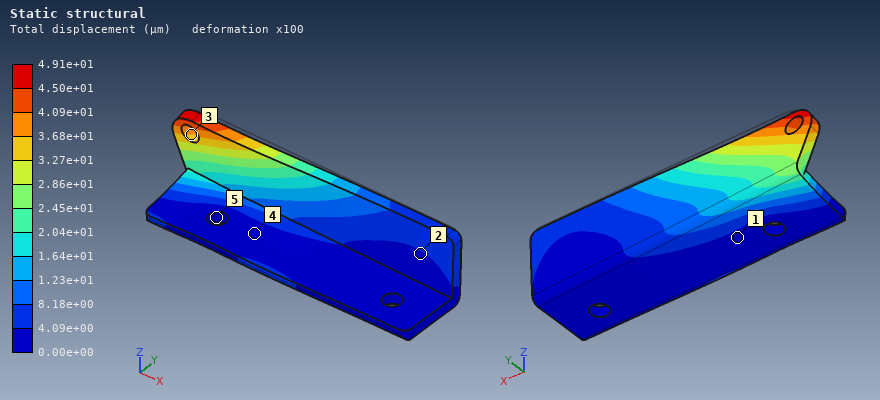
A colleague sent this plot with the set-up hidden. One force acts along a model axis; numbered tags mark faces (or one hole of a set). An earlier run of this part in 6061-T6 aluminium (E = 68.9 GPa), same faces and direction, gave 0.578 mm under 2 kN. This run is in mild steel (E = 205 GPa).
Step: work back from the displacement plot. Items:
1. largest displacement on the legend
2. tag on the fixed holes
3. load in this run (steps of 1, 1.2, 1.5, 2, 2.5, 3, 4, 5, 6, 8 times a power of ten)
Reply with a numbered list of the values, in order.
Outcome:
1. 4.91e+01 µm
2. 5
3. 500 N
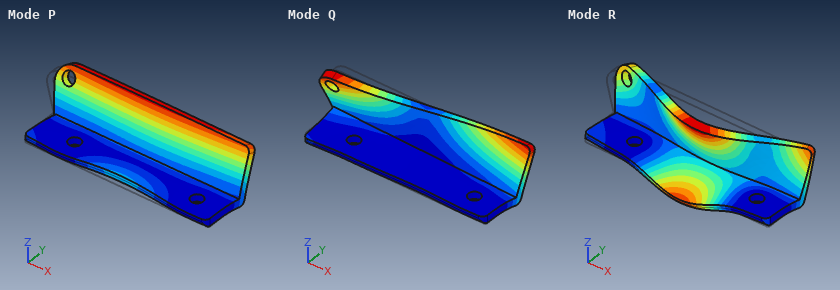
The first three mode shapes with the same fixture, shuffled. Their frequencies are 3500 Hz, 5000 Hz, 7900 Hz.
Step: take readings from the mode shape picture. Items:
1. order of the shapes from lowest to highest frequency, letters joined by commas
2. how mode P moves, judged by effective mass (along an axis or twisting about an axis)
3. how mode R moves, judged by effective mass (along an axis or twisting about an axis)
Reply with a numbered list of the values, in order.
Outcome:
1. P, Q, R
2. along Y
3. along Z
